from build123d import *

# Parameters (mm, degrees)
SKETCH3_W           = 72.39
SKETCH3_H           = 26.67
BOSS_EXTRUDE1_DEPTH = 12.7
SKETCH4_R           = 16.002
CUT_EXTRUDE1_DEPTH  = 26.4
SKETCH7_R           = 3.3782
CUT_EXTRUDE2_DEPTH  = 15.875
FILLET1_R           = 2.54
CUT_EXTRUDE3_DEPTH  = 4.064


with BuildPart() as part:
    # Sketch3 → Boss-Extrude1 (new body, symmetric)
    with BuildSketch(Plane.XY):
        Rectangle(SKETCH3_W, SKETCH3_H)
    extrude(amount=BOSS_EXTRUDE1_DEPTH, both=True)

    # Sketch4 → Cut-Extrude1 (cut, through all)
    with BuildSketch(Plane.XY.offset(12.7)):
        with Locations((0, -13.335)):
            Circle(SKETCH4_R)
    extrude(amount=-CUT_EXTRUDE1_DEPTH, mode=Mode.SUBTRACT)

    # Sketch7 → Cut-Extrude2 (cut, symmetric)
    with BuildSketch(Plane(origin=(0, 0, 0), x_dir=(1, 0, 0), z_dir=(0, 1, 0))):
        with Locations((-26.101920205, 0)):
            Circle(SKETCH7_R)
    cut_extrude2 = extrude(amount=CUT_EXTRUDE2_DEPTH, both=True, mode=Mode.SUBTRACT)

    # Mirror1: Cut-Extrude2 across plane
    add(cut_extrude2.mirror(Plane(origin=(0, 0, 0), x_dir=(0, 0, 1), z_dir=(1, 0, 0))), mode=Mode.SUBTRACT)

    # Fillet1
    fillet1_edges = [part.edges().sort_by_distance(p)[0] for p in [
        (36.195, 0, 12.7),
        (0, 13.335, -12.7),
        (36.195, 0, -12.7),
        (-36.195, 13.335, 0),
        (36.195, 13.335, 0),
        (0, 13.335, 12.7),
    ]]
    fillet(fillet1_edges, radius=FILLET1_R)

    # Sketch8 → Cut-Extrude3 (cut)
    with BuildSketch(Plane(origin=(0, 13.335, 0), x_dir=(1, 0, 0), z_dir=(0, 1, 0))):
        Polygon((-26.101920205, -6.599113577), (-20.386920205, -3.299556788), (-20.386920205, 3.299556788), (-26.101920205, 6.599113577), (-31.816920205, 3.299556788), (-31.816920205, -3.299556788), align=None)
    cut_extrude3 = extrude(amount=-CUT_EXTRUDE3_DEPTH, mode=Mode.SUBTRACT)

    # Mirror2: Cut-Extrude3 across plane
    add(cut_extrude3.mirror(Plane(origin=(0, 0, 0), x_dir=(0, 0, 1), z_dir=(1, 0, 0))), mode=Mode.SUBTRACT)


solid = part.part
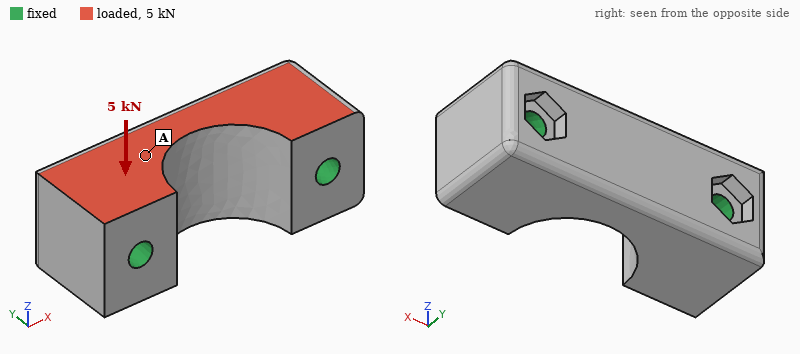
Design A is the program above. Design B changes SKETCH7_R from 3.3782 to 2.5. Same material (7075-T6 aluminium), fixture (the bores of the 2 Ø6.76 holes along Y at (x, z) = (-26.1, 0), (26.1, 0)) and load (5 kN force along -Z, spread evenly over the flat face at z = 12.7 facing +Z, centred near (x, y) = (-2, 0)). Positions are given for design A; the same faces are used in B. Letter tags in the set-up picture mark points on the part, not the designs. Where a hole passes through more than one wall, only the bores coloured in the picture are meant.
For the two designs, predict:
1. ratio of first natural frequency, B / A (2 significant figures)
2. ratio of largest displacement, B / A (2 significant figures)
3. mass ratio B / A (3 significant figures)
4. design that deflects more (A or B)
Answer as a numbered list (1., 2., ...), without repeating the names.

1. 0.87
2. 1.2
3. 1.02
4. B
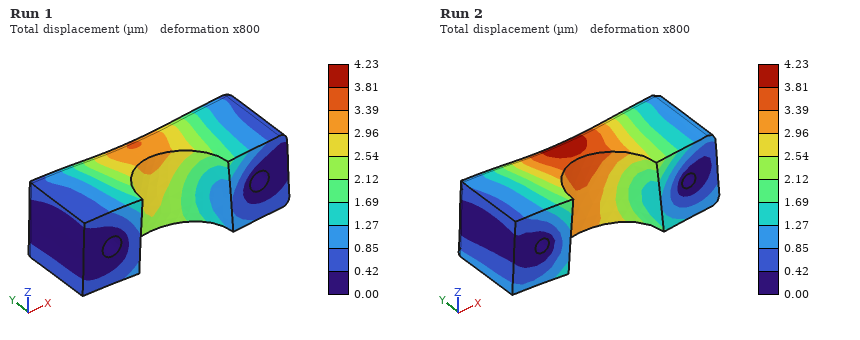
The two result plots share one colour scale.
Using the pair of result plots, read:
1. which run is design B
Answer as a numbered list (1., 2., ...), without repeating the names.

1. Run 2
